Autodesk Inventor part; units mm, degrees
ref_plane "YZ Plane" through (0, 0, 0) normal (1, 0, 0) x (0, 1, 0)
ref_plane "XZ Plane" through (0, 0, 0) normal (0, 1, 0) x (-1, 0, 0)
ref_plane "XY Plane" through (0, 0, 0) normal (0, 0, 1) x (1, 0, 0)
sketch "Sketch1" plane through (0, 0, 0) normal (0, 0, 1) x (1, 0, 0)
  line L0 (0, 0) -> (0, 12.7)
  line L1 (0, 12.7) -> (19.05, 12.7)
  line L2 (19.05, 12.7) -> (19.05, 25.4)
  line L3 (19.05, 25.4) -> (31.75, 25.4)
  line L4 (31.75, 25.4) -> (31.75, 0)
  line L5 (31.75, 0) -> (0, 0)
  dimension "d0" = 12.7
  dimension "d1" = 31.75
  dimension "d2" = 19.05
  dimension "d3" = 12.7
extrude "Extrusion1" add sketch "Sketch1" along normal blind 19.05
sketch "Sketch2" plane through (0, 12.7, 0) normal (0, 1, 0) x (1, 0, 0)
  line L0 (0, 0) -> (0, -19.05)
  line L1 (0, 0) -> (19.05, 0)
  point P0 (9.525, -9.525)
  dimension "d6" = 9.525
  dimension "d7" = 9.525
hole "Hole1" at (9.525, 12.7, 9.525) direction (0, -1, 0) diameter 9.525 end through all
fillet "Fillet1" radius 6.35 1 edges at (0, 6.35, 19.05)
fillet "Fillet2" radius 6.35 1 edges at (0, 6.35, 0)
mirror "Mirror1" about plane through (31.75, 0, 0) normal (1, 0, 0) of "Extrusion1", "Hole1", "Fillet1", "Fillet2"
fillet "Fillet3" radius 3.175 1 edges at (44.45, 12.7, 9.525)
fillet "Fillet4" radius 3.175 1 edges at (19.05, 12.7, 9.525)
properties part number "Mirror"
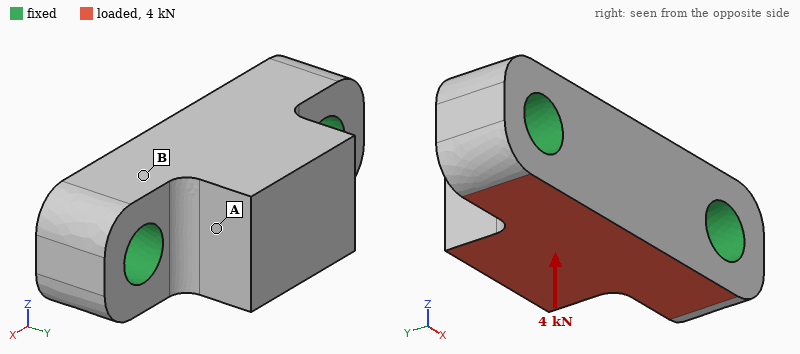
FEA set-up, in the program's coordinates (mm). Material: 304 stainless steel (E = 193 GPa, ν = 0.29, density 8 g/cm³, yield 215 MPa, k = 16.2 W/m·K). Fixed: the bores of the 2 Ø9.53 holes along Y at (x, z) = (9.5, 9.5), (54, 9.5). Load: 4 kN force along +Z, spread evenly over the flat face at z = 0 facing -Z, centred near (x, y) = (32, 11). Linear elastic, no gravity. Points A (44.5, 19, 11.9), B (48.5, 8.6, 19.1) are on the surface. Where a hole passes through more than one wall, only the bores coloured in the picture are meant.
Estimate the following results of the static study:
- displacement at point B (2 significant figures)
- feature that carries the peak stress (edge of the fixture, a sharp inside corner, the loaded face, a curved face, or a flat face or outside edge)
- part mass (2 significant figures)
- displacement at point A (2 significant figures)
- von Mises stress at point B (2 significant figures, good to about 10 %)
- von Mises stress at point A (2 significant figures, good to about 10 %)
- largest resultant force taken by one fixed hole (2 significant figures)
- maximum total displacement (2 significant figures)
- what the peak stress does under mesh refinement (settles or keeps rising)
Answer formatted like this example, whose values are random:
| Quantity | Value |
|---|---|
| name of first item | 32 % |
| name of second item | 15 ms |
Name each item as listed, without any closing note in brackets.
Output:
| Quantity | Value |
|---|---|
| displacement at point B | 0.84 µm |
| feature that carries the peak stress | edge of the fixture |
| part mass | 150 g |
| displacement at point A | 3.0 µm |
| von Mises stress at point B | 17 MPa |
| von Mises stress at point A | 8.2 MPa |
| largest resultant force taken by one fixed hole | 2.0 kN |
| maximum total displacement | 4.7 µm |
| what the peak stress does under mesh refinement | keeps rising |
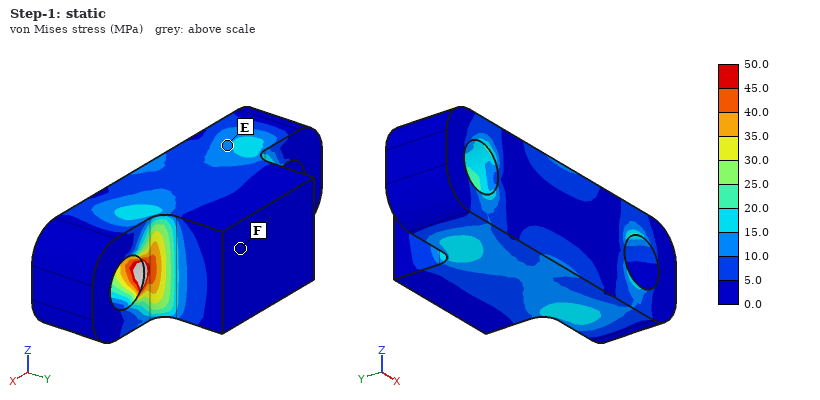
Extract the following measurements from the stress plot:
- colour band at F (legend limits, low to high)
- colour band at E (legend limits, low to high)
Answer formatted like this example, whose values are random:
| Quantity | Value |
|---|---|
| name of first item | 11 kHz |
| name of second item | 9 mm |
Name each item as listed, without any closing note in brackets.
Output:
| Quantity | Value |
|---|---|
| colour band at F | 0.0 to 5.0 MPa |
| colour band at E | 10.0 to 15.0 MPa |
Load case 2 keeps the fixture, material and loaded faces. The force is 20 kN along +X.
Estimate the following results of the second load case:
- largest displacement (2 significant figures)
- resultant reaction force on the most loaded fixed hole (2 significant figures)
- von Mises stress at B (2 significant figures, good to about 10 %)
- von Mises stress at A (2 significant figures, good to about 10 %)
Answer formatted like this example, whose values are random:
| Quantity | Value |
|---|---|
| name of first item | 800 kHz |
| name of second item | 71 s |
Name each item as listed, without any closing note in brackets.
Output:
| Quantity | Value |
|---|---|
| largest displacement | 11 µm |
| resultant reaction force on the most loaded fixed hole | 11 kN |
| von Mises stress at B | 23 MPa |
| von Mises stress at A | 22 MPa |
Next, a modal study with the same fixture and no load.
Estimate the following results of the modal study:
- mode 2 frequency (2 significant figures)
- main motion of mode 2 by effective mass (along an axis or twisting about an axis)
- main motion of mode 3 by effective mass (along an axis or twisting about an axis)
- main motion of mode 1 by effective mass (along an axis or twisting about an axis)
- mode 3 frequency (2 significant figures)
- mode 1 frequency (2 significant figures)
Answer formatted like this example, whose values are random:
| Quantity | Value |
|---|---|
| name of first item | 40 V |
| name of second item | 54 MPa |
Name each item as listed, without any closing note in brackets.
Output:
| Quantity | Value |
|---|---|
| mode 2 frequency | 24 kHz |
| main motion of mode 2 by effective mass | along Y |
| main motion of mode 3 by effective mass | along Z |
| main motion of mode 1 by effective mass | along Z |
| mode 3 frequency | 30 kHz |
| mode 1 frequency | 14 kHz |
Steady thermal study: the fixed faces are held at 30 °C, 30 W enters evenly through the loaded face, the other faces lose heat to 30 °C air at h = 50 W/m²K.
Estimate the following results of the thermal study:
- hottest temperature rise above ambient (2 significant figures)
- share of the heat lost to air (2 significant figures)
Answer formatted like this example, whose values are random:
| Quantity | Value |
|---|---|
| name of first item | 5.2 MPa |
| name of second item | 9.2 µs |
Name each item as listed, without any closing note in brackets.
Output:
| Quantity | Value |
|---|---|
| hottest temperature rise above ambient | 46 K |
| share of the heat lost to air | 11 % |
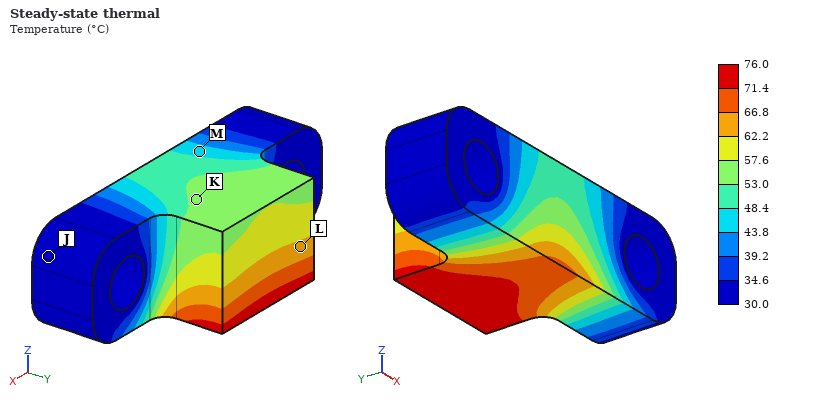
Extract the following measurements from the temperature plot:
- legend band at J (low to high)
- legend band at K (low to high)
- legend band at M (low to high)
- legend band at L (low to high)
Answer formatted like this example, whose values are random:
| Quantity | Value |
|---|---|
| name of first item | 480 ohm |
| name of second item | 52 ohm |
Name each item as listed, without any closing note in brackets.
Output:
| Quantity | Value |
|---|---|
| legend band at J | 30.0 to 34.6 °C |
| legend band at K | 53.0 to 57.6 °C |
| legend band at M | 43.8 to 48.4 °C |
| legend band at L | 62.2 to 66.8 °C |
